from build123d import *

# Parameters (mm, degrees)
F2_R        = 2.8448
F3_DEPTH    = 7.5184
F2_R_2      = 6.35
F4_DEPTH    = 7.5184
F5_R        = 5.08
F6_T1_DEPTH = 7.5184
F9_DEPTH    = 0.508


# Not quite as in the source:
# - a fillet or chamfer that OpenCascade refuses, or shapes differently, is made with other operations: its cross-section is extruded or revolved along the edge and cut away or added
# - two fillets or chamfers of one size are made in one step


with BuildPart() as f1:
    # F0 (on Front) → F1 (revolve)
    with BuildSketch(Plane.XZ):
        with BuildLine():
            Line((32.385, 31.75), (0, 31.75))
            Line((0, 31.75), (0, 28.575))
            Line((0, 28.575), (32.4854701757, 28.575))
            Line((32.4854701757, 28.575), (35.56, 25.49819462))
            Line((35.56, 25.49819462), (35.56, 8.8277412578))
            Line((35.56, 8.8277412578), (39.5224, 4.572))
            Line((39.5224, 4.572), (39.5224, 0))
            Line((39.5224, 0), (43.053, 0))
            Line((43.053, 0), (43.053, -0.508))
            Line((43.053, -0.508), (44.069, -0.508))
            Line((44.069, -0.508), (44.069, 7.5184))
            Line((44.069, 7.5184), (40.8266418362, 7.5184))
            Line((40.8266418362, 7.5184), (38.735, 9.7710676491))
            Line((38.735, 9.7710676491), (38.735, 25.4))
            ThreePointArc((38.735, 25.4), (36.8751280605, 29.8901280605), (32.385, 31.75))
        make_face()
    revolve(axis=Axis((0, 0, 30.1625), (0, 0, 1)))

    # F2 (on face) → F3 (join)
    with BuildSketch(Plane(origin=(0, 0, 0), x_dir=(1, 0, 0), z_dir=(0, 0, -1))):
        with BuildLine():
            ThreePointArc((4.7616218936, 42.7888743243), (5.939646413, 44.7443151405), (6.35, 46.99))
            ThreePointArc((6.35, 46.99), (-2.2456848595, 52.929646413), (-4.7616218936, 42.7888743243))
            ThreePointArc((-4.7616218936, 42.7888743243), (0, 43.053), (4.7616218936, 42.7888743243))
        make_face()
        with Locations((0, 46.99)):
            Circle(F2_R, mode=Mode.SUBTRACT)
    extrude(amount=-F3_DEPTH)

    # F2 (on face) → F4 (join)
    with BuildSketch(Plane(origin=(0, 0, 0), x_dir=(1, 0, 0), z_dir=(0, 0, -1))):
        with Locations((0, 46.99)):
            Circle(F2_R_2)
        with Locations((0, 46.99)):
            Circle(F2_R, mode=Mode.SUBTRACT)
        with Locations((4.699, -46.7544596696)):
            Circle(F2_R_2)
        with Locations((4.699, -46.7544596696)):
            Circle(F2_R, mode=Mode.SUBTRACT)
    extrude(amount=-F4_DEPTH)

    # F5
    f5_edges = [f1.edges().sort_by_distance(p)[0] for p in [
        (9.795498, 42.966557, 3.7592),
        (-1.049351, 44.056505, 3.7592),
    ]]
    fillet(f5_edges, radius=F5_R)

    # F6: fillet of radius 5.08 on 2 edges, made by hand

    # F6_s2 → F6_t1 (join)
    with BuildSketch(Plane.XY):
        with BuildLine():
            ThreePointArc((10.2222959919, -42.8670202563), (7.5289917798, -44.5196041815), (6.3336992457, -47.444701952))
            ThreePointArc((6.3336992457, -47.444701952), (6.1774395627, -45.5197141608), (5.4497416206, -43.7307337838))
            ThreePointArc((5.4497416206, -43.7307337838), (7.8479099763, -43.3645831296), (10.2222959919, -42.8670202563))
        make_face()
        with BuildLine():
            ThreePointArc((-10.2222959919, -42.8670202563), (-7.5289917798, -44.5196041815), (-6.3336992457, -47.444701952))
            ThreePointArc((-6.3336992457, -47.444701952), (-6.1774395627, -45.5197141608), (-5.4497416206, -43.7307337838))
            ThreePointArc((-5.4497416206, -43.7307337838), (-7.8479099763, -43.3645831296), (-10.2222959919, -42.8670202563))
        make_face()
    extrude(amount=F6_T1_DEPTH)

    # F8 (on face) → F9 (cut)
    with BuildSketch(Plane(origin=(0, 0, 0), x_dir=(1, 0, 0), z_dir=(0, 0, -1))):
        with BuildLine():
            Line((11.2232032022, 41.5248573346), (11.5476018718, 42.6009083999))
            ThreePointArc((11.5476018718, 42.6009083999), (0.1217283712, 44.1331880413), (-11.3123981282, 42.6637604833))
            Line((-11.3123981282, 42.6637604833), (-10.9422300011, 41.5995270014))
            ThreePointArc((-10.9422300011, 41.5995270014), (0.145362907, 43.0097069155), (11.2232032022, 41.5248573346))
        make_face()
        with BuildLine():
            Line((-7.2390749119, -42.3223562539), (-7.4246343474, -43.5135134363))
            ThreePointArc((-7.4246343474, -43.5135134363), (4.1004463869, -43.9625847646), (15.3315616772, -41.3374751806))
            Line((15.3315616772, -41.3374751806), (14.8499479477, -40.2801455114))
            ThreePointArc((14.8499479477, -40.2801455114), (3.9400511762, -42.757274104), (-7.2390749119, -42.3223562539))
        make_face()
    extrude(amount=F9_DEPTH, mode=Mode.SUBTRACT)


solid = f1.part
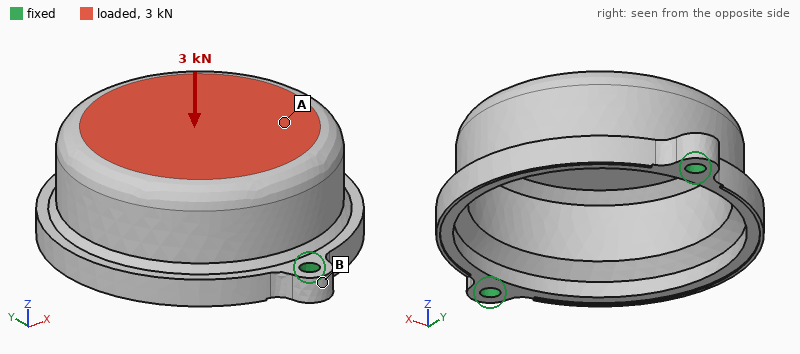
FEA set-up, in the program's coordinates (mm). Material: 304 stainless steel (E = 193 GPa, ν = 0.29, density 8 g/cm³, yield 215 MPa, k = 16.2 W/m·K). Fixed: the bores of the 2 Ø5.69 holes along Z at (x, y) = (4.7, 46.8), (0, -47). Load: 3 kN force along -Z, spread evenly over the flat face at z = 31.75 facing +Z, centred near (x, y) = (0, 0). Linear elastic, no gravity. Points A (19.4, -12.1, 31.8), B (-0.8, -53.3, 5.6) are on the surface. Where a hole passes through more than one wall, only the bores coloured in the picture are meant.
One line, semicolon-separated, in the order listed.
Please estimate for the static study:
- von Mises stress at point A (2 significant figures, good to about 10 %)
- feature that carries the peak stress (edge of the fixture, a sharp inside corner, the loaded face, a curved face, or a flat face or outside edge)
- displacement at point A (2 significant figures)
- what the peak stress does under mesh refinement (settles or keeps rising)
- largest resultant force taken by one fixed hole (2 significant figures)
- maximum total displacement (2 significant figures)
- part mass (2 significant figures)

33 MPa; edge of the fixture; 26 µm; keeps rising; 1.7 kN; 59 µm; 330 g
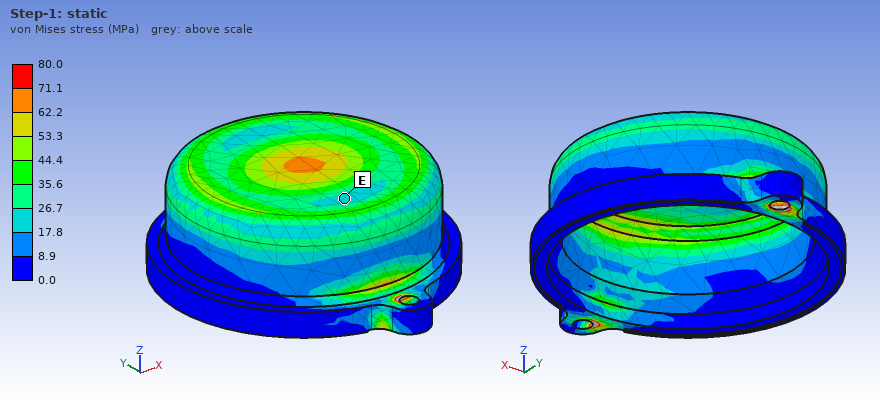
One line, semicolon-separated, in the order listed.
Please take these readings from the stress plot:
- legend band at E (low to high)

17.8 to 26.7 MPa
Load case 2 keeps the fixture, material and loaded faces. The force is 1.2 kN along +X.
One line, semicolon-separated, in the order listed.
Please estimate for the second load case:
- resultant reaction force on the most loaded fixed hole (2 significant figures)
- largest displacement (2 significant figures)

600 N; 56 µm
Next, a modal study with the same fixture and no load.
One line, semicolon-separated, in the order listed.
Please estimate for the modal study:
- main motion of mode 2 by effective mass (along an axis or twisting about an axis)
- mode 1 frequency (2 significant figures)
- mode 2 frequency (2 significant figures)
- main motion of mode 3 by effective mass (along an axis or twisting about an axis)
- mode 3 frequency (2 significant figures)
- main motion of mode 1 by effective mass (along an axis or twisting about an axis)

along Y; 1500 Hz; 3300 Hz; along Y; 3800 Hz; along X
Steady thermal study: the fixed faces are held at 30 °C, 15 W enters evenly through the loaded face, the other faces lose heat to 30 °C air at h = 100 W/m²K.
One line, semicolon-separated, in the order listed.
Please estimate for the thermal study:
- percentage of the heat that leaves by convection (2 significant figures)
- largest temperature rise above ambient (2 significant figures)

96 %; 25 K
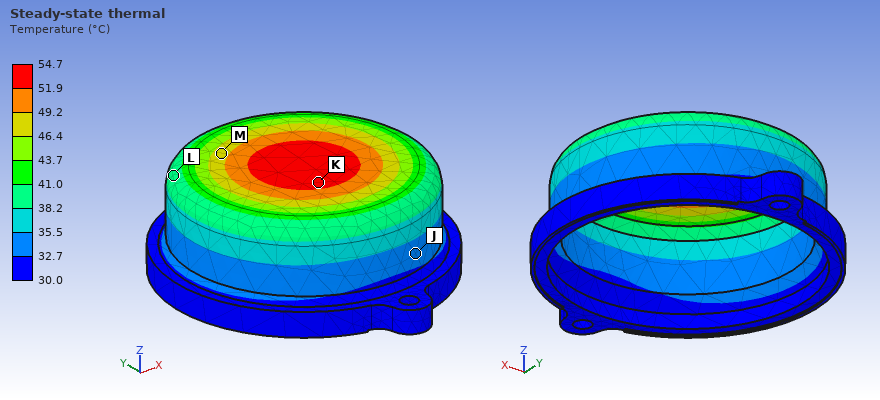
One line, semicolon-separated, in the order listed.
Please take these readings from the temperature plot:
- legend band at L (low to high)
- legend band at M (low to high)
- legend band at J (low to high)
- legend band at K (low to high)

38.2 to 41.0 °C; 46.4 to 49.2 °C; 32.7 to 35.5 °C; 51.9 to 54.7 °C
